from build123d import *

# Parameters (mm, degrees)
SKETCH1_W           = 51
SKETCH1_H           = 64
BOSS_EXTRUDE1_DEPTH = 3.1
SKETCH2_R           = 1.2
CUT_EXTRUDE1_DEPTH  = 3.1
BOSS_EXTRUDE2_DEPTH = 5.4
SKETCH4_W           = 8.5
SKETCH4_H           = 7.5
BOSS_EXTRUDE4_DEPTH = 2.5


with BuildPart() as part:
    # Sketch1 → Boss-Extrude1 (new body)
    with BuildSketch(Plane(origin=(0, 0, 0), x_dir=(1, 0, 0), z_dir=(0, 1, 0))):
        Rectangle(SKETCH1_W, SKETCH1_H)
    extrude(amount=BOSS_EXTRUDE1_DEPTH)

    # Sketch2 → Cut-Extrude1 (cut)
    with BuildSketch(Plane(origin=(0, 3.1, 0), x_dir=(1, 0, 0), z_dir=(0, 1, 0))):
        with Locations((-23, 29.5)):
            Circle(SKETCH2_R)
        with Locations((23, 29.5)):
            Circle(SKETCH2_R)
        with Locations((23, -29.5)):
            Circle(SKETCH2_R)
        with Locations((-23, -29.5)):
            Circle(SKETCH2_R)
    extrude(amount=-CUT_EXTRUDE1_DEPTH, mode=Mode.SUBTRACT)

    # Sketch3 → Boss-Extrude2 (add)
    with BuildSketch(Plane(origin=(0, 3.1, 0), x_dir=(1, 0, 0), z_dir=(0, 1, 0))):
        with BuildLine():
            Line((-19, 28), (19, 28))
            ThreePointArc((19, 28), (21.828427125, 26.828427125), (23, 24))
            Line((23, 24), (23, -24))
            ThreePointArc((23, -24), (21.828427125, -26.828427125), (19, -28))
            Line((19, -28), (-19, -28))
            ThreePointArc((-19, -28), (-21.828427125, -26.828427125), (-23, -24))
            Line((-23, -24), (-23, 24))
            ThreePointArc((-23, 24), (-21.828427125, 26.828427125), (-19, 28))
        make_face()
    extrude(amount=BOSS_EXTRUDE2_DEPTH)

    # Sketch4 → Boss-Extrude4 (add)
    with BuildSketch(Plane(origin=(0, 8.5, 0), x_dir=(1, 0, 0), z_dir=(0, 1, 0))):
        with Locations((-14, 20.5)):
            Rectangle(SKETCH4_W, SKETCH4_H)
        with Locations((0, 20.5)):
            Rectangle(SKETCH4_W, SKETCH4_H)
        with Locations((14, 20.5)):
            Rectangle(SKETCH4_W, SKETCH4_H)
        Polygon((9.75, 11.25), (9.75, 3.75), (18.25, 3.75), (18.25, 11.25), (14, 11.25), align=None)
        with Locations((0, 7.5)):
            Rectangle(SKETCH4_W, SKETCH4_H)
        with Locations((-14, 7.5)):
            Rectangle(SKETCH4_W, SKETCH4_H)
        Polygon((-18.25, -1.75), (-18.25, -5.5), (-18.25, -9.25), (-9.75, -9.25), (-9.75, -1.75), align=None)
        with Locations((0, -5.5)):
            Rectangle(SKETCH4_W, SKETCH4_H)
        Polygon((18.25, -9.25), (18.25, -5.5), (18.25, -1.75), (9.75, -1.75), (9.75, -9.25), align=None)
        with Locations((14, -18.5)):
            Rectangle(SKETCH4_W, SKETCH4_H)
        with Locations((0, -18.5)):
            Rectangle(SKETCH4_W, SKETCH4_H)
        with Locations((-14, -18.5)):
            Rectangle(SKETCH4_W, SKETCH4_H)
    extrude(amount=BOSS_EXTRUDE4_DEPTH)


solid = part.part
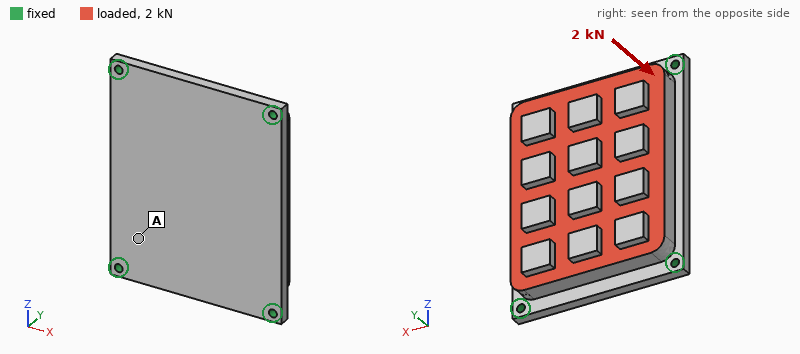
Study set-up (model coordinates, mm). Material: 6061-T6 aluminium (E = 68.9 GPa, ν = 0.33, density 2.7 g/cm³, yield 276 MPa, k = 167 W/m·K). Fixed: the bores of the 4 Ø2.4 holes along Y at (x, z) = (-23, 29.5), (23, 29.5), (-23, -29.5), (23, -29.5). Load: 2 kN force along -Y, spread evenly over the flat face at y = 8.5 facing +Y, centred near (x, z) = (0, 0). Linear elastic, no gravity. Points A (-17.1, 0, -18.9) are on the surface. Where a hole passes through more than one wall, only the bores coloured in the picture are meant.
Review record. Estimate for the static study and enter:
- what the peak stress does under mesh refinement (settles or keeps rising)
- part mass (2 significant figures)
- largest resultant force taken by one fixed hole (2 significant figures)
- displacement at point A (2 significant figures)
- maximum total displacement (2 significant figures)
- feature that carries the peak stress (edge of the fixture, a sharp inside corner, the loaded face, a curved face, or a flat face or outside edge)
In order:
keeps rising
70 g
750 N
17 µm
27 µm
edge of the fixture
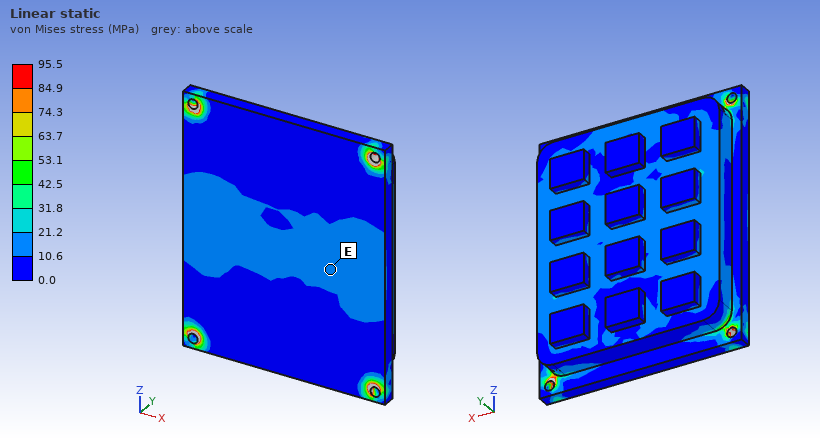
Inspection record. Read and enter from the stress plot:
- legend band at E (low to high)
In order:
10.6 to 21.2 MPa
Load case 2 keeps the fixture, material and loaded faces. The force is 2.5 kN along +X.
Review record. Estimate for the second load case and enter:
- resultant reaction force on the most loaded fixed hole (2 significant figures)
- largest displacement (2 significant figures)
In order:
740 N
8.7 µm
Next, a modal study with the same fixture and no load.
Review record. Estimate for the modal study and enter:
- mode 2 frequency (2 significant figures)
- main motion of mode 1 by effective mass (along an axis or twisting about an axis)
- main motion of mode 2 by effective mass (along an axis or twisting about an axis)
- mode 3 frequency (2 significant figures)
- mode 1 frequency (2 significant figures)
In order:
9800 Hz
along Y
twisting about Z
11 kHz
5800 Hz
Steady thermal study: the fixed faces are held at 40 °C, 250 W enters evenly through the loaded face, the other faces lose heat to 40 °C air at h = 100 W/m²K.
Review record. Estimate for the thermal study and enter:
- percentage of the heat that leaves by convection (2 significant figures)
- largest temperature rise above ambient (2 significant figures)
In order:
20 %
82 K
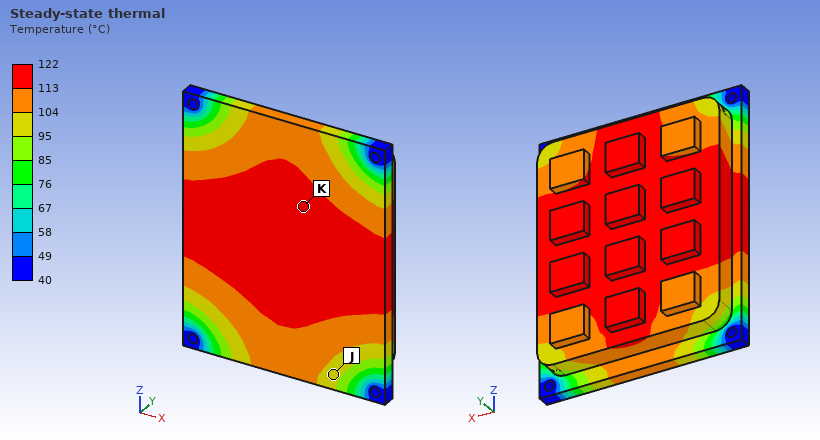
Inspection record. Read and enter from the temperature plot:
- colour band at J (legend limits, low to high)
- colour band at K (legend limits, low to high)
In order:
95 to 104 °C
113 to 122 °C
